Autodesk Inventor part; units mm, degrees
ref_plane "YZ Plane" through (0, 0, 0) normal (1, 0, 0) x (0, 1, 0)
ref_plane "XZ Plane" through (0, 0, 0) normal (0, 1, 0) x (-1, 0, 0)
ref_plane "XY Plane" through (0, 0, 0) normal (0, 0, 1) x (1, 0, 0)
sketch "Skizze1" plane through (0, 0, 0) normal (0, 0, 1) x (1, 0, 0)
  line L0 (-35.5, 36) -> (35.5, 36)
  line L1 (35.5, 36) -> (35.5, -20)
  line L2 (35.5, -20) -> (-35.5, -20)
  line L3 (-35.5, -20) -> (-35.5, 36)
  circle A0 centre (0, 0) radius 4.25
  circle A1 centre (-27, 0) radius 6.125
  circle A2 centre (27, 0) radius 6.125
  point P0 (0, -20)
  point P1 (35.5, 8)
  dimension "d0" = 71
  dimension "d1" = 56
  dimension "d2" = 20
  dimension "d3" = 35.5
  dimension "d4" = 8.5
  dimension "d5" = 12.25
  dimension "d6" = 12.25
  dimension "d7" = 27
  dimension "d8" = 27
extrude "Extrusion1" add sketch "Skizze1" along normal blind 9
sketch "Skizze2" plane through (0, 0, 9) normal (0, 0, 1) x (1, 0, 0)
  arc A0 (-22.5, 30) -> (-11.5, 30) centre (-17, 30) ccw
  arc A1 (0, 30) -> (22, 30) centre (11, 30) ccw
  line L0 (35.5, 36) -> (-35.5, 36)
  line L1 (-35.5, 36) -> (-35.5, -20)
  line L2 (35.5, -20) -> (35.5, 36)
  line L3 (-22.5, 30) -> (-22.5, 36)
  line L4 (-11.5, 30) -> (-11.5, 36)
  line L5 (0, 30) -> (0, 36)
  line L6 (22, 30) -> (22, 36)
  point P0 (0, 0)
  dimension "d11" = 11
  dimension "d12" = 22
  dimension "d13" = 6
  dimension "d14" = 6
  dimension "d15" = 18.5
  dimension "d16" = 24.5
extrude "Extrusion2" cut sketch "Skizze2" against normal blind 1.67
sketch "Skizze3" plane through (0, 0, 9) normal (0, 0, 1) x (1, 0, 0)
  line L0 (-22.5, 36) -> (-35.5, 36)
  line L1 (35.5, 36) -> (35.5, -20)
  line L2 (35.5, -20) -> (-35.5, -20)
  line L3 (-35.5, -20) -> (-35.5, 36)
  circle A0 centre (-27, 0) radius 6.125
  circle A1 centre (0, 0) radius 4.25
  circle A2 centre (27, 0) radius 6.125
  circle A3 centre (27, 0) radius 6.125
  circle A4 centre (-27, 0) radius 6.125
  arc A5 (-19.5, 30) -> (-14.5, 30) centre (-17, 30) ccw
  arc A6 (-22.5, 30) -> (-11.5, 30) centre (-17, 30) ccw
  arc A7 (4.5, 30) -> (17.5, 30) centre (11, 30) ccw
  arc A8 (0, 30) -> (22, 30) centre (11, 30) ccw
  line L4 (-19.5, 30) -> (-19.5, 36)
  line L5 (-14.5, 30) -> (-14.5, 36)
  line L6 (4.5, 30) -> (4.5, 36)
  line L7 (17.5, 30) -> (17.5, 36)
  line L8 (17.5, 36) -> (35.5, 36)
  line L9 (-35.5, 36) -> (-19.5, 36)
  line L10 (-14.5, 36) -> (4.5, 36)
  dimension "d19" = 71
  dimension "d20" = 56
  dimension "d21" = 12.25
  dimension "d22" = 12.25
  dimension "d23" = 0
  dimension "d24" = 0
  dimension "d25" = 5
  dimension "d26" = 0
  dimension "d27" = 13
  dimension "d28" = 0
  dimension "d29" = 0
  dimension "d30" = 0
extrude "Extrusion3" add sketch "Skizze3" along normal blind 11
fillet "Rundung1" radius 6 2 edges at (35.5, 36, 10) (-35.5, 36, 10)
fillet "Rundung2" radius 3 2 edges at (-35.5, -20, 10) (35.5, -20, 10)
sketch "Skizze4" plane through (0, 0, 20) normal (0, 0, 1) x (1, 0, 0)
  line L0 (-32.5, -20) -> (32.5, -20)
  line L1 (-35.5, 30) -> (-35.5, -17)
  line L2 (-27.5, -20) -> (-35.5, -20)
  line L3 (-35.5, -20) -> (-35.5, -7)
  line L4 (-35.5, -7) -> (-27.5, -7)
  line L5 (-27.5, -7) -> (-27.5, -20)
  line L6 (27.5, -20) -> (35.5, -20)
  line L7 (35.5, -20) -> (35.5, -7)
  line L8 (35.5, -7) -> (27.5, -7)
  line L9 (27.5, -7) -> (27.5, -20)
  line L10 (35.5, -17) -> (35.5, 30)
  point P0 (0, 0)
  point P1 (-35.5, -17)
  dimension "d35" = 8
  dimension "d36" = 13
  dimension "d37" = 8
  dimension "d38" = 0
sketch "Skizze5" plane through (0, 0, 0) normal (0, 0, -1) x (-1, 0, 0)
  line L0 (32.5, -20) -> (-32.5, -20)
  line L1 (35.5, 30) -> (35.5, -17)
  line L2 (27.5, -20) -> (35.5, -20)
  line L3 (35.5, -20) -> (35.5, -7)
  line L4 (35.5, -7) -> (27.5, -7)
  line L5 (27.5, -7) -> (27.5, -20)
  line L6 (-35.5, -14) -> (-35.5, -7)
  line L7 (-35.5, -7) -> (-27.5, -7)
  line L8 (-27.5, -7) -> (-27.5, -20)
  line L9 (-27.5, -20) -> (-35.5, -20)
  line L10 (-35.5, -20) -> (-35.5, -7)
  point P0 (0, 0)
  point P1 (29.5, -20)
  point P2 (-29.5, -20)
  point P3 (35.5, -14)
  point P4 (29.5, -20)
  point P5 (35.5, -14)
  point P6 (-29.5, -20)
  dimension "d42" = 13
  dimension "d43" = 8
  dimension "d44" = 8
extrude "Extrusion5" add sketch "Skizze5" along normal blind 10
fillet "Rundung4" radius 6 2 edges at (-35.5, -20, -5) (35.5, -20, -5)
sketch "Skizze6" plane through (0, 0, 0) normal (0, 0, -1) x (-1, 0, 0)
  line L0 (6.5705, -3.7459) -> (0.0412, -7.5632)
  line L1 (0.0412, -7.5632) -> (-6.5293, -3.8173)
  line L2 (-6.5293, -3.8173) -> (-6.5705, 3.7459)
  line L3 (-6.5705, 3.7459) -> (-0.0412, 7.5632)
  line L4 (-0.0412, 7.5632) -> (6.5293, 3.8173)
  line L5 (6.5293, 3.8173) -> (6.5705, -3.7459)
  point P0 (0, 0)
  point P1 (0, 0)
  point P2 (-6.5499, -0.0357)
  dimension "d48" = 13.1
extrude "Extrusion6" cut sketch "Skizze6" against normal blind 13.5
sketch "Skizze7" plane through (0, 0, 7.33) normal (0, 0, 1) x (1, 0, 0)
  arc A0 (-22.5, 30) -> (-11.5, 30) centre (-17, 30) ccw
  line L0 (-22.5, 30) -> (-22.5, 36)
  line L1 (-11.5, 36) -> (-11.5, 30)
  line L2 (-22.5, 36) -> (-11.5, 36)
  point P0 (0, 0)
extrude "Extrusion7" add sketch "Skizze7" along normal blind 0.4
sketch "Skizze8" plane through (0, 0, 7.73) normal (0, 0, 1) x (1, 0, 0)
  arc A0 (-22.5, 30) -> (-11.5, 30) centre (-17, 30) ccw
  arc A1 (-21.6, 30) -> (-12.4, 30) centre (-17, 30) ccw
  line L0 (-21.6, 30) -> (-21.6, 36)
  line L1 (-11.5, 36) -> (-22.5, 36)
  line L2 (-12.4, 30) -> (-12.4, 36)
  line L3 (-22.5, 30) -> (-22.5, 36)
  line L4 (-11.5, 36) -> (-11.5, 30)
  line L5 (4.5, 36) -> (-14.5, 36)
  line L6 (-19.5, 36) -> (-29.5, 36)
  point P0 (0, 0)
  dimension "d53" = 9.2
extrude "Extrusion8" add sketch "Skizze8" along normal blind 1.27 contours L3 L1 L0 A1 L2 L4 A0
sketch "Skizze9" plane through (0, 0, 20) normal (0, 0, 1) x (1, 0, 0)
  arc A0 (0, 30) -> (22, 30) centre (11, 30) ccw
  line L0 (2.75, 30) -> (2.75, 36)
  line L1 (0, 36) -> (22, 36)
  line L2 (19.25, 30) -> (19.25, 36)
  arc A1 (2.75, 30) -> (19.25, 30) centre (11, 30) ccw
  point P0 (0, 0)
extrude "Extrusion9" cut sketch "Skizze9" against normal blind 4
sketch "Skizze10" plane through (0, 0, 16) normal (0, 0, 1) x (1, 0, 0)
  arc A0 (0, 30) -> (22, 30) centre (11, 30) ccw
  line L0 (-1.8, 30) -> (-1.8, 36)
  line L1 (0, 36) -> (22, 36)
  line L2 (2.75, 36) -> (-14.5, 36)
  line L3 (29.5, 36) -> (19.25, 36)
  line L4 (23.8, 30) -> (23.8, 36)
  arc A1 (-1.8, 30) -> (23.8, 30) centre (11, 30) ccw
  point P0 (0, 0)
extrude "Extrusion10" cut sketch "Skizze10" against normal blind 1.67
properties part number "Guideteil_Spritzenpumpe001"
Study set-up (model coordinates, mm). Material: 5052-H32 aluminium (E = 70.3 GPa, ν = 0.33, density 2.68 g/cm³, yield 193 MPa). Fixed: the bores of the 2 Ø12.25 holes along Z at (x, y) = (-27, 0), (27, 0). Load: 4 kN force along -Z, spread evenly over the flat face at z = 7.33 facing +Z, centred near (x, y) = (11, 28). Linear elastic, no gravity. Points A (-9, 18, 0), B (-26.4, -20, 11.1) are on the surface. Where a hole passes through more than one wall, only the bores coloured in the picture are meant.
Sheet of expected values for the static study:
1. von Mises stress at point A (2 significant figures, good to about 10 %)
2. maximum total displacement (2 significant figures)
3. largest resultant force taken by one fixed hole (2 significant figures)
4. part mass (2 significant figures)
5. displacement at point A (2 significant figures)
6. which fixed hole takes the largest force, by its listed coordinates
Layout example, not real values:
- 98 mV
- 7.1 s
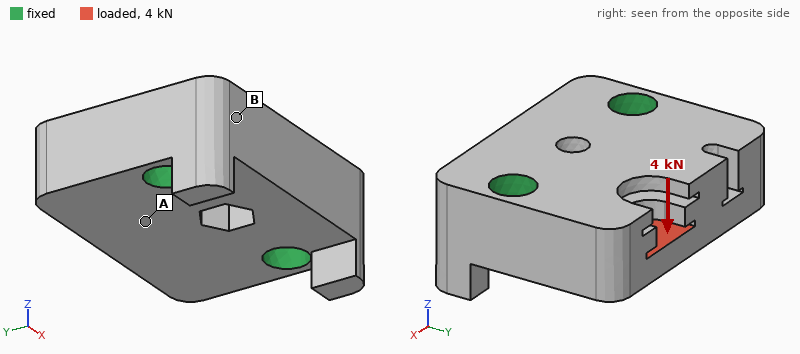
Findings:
- 16 MPa
- 40 µm
- 2.9 kN
- 190 g
- 9.8 µm
- (27, 0)
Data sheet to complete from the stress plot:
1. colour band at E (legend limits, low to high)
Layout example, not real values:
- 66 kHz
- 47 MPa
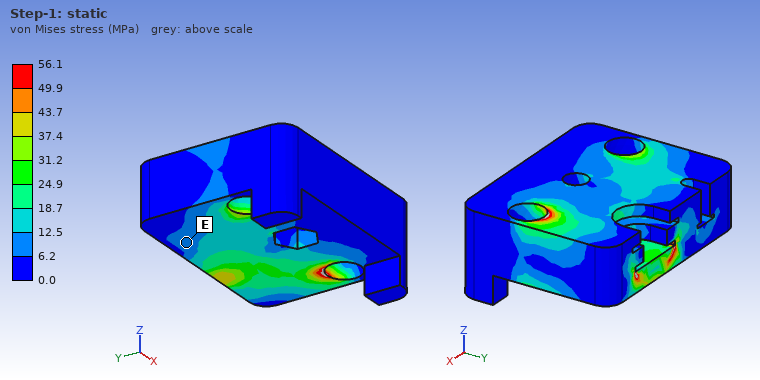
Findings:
- 6.2 to 12.5 MPa
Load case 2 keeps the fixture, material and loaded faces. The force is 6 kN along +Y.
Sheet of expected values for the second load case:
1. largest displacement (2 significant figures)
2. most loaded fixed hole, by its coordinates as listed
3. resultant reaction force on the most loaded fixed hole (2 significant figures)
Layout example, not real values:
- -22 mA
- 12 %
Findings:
- 18 µm
- (27, 0)
- 4.4 kN
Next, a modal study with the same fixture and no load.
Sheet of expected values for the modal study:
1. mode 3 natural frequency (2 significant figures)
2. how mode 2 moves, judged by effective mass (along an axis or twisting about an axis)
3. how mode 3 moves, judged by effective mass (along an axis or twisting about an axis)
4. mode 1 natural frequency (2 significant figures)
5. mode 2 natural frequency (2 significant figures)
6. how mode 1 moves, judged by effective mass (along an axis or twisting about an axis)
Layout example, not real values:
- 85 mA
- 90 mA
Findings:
- 20 kHz
- twisting about Y
- along X
- 11 kHz
- 16 kHz
- along Z
